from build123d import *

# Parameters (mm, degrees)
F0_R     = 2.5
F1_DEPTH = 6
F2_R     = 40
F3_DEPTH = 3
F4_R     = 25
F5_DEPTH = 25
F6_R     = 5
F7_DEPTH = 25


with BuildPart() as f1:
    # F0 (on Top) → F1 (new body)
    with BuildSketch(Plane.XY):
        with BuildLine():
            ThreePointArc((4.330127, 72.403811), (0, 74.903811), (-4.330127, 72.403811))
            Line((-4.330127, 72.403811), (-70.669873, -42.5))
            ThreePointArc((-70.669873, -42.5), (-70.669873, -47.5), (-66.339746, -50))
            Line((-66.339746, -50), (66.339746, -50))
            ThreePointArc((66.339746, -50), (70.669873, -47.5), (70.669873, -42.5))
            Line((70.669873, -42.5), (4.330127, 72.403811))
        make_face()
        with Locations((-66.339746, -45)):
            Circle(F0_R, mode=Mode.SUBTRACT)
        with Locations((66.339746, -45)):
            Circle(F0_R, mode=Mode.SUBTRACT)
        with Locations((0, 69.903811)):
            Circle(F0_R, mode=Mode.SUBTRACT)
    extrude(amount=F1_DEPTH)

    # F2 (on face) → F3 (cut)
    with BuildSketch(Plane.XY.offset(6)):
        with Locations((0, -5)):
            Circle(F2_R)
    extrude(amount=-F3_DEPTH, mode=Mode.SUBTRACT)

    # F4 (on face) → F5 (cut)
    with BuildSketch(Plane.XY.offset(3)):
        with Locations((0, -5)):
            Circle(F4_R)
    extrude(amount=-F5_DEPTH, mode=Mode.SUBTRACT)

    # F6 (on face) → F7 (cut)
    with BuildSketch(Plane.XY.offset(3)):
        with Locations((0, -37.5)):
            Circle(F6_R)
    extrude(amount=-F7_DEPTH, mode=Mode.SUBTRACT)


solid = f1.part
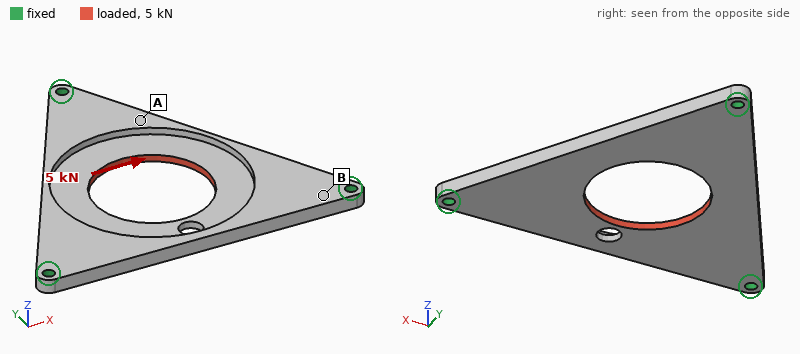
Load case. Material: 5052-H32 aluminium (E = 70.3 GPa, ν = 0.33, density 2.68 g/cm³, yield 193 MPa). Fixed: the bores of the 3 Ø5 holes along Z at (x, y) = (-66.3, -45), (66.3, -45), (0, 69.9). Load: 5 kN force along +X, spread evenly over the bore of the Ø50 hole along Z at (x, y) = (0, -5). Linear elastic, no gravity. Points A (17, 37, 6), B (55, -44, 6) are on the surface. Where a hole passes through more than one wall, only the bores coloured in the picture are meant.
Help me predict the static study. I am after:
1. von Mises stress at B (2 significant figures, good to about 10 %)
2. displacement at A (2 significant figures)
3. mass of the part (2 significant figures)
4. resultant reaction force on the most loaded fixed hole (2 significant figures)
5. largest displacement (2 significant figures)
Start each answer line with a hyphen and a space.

- 21 MPa
- 54 µm
- 98 g
- 2.2 kN
- 74 µm
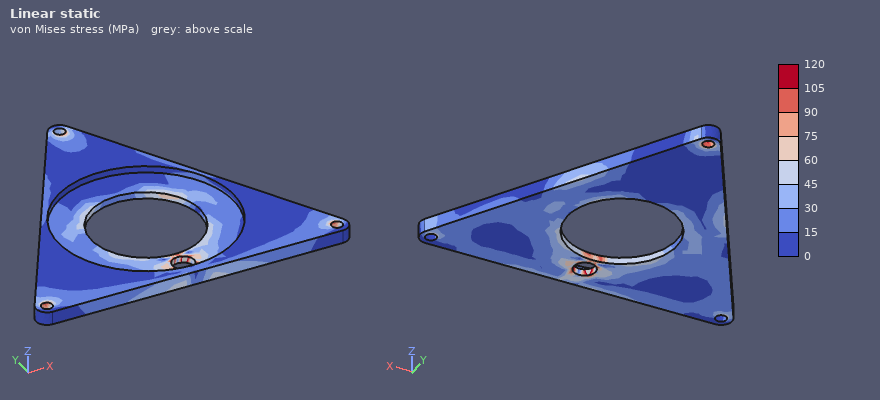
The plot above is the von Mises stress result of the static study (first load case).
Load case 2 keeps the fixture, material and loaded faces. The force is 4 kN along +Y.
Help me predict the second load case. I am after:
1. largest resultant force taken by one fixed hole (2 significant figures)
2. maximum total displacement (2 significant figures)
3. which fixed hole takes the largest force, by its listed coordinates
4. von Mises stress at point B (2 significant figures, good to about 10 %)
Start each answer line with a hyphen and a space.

- 2.0 kN
- 62 µm
- (0, 69.9)
- 12 MPa
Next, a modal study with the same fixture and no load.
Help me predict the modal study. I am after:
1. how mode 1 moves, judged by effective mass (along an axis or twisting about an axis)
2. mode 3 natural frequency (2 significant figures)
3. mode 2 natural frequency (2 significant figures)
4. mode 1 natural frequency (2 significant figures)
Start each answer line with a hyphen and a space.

- along Z
- 2100 Hz
- 2100 Hz
- 1500 Hz
